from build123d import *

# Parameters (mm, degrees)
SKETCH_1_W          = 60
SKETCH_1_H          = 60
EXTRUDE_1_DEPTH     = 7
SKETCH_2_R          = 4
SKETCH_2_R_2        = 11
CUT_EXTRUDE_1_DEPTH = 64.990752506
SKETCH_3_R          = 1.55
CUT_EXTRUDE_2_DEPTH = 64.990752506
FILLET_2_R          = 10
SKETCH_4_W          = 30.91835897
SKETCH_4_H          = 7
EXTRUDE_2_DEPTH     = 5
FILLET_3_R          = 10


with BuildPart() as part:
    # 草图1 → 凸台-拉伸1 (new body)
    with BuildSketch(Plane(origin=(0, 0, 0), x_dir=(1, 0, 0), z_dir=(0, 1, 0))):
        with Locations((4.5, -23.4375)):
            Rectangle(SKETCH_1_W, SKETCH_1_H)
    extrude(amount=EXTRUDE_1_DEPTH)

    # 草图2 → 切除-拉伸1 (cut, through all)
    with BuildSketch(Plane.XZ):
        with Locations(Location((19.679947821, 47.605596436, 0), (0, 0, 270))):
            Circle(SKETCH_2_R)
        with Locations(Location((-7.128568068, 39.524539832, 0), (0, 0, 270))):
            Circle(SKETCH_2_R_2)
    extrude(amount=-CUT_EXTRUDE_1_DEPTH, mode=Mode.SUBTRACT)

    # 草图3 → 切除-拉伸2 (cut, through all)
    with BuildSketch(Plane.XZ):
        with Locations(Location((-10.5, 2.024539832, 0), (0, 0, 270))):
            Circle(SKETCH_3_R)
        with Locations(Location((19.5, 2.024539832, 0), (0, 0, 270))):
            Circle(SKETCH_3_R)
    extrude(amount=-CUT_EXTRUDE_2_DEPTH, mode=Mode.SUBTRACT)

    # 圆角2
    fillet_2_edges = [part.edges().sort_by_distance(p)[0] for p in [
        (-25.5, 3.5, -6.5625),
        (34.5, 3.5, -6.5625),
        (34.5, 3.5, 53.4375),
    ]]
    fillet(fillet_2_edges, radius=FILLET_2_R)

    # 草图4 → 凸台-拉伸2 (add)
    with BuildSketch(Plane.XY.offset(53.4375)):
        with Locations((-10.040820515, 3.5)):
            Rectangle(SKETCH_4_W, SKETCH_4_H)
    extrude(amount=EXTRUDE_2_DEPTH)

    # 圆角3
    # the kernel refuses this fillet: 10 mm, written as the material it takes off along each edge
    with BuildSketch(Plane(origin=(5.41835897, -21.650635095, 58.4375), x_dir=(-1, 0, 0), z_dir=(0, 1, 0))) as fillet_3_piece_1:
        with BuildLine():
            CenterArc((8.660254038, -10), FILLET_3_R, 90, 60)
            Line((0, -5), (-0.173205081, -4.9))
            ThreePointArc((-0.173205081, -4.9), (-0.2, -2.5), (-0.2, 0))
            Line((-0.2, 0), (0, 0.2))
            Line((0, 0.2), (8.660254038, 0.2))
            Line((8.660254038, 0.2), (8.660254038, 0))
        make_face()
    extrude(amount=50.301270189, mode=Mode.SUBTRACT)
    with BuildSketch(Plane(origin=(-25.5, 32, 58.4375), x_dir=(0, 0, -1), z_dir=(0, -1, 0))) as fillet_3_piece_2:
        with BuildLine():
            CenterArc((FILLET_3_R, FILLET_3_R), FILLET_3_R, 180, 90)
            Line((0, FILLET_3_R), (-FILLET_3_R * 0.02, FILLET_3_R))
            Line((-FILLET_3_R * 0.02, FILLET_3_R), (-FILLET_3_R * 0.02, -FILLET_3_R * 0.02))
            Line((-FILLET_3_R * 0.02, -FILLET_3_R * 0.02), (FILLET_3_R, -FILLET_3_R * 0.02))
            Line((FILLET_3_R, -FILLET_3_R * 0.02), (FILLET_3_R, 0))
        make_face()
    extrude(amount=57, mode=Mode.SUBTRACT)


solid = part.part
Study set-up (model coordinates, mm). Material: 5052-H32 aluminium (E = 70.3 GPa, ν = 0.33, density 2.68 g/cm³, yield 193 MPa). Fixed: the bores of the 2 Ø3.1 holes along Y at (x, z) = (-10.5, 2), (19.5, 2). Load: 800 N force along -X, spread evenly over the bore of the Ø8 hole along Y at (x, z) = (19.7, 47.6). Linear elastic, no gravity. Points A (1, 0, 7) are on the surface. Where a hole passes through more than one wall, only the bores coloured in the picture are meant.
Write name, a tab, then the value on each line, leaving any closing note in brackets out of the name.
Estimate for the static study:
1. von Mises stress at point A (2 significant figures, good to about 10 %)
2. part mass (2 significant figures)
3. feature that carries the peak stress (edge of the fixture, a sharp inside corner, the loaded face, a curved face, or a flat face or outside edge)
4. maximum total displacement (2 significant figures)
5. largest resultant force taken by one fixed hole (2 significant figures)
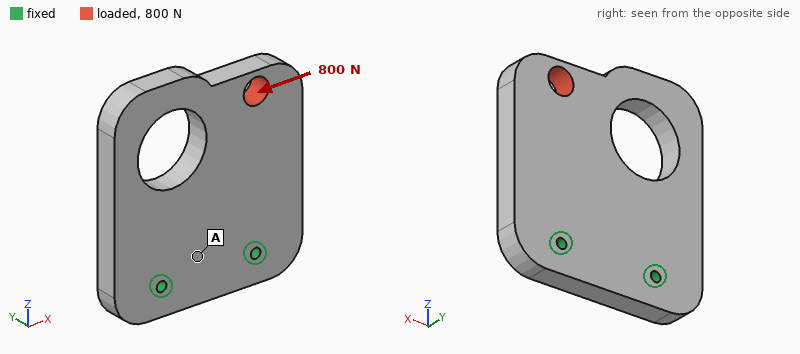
von Mises stress at point A	7.5 MPa
part mass	60 g
feature that carries the peak stress	edge of the fixture
maximum total displacement	19 µm
largest resultant force taken by one fixed hole	1.2 kN
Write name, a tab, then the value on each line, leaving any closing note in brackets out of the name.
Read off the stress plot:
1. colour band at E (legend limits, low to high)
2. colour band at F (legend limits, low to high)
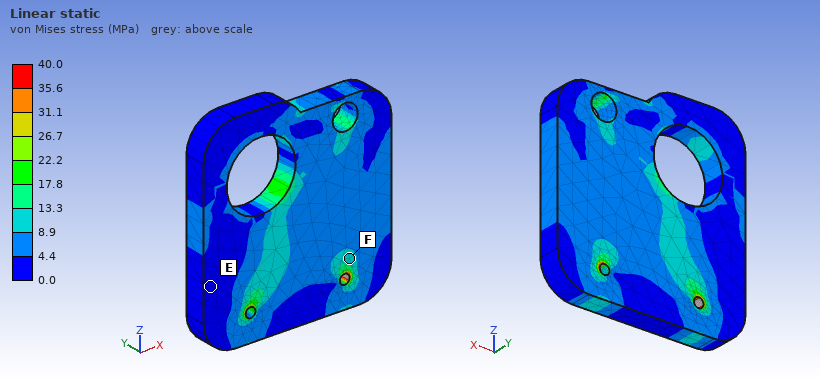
colour band at E	0.0 to 4.4 MPa
colour band at F	8.9 to 13.3 MPa
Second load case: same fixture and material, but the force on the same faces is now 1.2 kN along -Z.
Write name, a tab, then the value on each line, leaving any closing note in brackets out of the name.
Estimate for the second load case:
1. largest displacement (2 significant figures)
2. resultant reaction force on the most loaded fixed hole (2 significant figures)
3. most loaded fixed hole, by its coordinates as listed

largest displacement	9.8 µm
resultant reaction force on the most loaded fixed hole	1.2 kN
most loaded fixed hole, by its coordinates as listed	(19.5, 2)
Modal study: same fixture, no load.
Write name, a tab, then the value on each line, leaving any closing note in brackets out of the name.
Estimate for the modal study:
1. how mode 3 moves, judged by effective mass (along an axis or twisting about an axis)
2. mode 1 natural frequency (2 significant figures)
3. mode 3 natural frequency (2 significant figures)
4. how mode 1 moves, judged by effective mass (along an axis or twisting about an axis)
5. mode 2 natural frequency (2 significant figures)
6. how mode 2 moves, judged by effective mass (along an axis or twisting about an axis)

how mode 3 moves, judged by effective mass	along X
mode 1 natural frequency	2000 Hz
mode 3 natural frequency	7700 Hz
how mode 1 moves, judged by effective mass	along Y
mode 2 natural frequency	4000 Hz
how mode 2 moves, judged by effective mass	twisting about Z
